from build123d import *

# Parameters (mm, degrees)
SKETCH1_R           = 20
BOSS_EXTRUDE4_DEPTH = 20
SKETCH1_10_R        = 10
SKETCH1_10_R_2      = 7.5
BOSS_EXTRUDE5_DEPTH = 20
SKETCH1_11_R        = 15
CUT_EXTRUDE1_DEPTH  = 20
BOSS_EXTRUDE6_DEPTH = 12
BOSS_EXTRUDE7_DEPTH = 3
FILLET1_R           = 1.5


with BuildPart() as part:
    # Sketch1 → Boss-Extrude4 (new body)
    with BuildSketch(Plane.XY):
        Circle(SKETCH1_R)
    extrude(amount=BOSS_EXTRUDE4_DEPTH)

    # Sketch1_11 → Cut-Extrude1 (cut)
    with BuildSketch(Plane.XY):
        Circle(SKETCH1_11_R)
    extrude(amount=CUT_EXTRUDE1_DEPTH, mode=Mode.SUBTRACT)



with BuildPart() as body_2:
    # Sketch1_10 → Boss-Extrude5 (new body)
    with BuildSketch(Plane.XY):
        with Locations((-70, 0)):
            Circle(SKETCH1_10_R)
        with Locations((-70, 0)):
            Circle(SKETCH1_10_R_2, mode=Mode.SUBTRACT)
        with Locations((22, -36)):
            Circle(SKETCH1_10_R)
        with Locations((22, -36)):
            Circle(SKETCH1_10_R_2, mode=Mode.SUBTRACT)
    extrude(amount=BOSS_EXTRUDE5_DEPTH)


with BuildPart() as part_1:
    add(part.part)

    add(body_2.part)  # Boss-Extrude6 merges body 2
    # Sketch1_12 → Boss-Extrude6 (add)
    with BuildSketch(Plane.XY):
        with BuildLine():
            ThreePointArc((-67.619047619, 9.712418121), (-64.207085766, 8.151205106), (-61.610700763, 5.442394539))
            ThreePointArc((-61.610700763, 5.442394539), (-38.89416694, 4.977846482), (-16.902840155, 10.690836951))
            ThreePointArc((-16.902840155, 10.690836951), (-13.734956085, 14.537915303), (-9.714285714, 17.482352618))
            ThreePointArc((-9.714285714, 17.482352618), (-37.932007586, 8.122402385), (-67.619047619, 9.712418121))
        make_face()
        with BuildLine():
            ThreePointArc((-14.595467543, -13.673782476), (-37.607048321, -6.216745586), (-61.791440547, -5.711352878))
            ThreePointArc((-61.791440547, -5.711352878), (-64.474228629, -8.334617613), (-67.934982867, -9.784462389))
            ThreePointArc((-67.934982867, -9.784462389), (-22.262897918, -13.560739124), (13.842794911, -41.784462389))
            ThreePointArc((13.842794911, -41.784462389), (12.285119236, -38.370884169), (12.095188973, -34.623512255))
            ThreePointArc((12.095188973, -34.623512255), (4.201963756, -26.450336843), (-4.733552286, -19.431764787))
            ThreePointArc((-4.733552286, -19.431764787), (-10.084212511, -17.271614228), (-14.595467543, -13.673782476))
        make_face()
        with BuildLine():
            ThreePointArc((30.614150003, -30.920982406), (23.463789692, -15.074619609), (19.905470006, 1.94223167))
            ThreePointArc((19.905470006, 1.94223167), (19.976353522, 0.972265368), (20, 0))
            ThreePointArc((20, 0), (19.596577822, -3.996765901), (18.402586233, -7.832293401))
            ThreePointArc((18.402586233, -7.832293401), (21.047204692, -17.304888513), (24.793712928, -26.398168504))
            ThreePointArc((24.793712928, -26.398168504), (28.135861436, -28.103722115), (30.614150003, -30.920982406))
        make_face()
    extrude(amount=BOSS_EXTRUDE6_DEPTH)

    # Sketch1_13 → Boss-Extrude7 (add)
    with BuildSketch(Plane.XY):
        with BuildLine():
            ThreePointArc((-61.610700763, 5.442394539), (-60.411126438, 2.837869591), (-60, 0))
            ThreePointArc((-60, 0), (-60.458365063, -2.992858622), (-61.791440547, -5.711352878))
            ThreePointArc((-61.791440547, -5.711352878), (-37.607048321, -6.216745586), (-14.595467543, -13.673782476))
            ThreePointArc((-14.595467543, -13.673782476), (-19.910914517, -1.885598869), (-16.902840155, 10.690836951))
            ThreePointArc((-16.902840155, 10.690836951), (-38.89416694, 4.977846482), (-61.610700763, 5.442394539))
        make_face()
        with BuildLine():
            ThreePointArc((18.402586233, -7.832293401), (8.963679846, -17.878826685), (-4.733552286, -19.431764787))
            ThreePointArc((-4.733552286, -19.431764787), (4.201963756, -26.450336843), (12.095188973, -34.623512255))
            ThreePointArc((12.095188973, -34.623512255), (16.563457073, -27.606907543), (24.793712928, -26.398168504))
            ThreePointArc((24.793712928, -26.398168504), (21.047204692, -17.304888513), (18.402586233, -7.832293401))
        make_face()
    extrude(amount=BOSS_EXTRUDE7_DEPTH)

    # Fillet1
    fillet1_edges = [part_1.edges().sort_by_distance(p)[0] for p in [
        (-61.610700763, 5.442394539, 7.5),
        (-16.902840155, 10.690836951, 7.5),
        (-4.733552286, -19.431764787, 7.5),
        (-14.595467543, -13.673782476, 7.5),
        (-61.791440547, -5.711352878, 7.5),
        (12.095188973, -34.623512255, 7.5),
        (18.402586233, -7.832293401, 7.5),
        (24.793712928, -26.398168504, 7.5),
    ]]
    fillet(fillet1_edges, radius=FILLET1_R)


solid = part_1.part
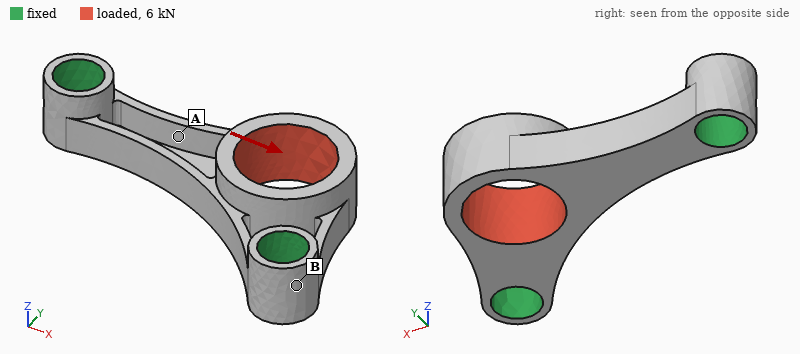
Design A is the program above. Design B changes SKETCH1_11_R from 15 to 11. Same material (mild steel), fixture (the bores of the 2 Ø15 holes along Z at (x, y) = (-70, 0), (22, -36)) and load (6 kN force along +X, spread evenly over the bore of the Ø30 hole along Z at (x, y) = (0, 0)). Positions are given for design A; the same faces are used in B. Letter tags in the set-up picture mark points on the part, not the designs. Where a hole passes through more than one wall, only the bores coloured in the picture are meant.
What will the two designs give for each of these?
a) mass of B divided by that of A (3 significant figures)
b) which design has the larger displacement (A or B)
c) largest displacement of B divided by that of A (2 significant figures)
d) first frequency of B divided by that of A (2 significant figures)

1.26
A
0.81
0.89
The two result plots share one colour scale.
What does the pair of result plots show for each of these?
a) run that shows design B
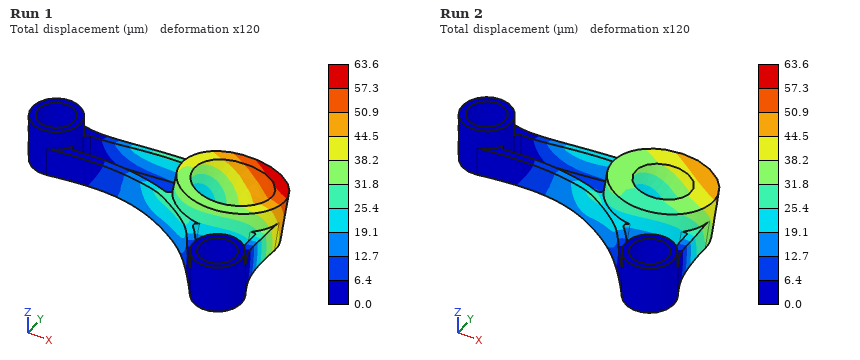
Run 2
